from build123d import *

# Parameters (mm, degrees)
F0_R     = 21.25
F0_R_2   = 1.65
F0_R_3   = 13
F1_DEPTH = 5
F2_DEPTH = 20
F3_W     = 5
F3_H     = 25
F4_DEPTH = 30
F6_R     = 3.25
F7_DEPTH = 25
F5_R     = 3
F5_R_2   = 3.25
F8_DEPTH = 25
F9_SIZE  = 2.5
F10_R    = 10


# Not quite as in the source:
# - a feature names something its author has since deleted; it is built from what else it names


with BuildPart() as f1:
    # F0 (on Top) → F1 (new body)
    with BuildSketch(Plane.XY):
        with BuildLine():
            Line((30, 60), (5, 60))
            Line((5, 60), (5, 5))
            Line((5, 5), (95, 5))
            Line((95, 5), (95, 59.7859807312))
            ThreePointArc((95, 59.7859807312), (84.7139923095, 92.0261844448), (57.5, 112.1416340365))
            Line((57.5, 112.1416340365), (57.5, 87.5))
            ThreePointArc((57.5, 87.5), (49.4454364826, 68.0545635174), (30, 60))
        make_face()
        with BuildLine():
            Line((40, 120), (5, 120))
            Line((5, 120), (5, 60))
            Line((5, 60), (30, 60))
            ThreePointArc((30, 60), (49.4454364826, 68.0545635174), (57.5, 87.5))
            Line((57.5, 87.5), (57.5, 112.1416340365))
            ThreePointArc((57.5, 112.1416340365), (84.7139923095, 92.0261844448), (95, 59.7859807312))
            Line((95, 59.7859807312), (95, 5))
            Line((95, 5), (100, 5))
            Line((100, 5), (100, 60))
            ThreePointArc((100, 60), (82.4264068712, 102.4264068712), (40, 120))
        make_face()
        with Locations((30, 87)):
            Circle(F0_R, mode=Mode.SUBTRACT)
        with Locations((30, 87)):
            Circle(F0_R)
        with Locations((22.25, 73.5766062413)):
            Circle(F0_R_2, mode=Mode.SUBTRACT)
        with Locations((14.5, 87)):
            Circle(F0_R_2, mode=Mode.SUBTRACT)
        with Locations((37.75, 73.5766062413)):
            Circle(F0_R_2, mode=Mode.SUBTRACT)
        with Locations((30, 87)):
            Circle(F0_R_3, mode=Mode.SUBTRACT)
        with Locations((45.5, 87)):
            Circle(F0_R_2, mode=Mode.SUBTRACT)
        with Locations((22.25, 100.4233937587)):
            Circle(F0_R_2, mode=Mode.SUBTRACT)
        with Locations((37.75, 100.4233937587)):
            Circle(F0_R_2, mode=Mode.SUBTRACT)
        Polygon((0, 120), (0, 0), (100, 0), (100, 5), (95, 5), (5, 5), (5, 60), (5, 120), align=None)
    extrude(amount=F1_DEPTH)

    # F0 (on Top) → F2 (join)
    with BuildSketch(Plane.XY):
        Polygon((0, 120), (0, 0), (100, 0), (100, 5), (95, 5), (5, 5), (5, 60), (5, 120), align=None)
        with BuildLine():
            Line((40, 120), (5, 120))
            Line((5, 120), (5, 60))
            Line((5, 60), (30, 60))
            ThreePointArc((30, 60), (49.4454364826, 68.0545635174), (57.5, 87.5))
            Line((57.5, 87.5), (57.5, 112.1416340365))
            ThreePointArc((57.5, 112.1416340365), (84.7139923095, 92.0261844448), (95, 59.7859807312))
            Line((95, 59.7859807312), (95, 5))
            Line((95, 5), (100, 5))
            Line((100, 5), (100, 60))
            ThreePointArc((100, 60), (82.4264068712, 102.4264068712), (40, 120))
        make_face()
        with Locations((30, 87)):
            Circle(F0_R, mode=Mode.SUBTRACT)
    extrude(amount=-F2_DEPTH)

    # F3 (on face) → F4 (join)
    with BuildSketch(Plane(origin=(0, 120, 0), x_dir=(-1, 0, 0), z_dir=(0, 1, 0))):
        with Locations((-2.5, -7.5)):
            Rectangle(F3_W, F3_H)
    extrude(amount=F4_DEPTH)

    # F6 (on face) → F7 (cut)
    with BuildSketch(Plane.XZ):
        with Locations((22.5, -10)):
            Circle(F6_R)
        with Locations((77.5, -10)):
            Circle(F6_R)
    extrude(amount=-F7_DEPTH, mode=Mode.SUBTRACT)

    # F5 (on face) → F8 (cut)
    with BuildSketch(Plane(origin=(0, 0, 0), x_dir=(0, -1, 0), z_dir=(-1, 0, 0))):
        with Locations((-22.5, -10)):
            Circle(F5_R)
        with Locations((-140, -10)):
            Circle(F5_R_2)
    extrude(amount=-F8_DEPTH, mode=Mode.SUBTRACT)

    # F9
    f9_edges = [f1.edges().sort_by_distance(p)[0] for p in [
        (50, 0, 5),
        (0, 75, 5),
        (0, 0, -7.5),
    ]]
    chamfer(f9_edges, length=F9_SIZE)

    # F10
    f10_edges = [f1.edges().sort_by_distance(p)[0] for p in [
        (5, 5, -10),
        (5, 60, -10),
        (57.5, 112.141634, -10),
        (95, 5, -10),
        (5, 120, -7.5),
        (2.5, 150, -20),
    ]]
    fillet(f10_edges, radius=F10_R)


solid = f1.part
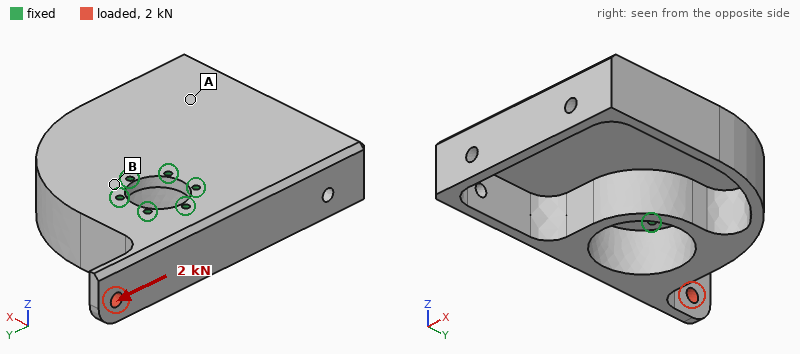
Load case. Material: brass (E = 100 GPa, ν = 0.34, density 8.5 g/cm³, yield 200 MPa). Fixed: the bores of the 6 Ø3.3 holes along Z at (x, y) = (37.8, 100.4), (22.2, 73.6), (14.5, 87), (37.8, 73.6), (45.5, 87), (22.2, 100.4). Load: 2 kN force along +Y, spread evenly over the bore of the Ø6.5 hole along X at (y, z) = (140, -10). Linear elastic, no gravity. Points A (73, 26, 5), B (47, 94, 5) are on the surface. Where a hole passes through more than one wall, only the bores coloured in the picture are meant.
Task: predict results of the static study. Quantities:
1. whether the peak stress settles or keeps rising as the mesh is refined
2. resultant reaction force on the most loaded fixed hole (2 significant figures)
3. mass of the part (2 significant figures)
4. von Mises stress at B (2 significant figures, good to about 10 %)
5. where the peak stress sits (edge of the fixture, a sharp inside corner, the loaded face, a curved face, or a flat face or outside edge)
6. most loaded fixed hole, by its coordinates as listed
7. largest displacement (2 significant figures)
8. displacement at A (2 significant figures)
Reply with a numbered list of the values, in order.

1. keeps rising
2. 1.3 kN
3. 1.1 kg
4. 5.9 MPa
5. edge of the fixture
6. (14.5, 87)
7. 35 µm
8. 13 µm
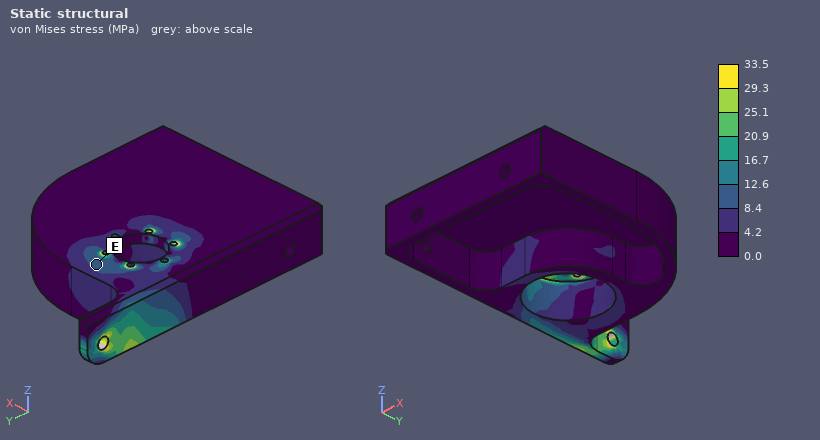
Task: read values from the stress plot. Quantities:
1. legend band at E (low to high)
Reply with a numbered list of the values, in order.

1. 8.4 to 12.6 MPa
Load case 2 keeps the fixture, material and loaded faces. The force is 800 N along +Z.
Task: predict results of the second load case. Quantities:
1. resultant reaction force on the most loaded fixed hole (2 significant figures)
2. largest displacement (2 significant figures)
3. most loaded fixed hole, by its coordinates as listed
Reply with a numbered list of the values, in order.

1. 1.3 kN
2. 61 µm
3. (22.2, 100.4)
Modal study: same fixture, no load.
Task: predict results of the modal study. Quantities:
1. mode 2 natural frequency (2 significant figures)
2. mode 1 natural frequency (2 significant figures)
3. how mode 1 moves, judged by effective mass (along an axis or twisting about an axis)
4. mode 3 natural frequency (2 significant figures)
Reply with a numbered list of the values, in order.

1. 1200 Hz
2. 580 Hz
3. along Z
4. 1900 Hz
